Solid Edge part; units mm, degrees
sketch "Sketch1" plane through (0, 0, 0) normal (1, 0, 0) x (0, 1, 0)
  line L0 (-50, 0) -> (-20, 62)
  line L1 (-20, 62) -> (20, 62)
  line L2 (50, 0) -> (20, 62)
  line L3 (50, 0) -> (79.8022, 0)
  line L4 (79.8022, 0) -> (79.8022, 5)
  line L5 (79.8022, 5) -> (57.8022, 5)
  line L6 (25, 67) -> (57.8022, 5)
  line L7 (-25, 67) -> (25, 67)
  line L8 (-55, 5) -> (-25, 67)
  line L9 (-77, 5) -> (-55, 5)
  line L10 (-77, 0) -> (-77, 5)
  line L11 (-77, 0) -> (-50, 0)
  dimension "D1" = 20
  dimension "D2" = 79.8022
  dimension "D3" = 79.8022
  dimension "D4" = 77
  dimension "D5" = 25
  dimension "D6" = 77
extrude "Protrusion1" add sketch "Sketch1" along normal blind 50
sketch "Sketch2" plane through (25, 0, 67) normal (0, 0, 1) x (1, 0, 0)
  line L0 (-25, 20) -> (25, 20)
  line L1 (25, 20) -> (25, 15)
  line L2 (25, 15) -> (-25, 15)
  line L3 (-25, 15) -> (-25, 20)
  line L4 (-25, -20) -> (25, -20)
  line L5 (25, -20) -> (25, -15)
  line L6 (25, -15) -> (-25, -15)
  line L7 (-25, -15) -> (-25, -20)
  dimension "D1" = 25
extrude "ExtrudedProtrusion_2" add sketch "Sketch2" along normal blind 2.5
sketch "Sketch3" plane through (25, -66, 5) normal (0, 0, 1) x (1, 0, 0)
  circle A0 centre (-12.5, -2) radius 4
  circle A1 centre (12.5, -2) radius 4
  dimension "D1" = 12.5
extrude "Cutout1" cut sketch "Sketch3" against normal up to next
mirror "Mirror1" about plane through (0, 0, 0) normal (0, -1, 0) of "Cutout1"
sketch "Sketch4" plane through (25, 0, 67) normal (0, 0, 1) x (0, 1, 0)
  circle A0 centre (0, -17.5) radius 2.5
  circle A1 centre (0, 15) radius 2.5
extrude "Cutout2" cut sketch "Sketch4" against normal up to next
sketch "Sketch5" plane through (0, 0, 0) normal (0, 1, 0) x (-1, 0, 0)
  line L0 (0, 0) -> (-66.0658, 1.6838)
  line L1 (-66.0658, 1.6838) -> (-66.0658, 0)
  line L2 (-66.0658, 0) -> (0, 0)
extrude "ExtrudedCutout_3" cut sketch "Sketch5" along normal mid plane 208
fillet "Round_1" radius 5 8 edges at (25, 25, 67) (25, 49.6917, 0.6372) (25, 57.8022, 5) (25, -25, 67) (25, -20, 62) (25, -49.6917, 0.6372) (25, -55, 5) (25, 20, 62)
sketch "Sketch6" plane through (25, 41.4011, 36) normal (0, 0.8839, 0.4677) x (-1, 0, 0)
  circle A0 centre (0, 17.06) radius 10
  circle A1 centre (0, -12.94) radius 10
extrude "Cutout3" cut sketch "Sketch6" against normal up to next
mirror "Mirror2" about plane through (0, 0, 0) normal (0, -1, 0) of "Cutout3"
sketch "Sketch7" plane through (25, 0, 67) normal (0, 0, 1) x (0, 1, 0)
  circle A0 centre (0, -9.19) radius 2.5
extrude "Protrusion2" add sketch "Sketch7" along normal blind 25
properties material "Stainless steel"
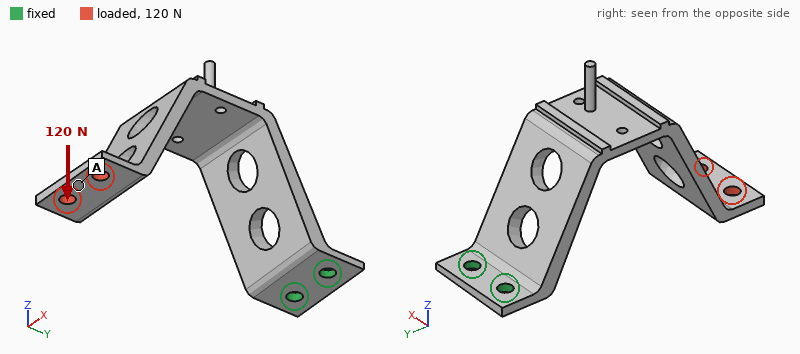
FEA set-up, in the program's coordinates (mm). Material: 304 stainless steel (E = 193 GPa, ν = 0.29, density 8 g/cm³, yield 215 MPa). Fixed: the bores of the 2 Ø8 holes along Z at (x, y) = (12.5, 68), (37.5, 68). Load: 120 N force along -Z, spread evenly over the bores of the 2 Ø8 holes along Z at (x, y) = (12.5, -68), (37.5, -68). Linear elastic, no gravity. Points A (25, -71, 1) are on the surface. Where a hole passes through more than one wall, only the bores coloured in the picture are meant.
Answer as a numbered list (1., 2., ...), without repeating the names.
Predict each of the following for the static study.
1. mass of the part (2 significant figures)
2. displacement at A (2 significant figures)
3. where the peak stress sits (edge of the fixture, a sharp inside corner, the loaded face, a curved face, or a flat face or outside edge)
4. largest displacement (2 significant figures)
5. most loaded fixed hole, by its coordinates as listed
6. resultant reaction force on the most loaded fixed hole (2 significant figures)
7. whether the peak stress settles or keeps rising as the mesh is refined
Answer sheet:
1. 510 g
2. 0.96 mm
3. edge of the fixture
4. 1.0 mm
5. (12.5, 68)
6. 100 N
7. keeps rising
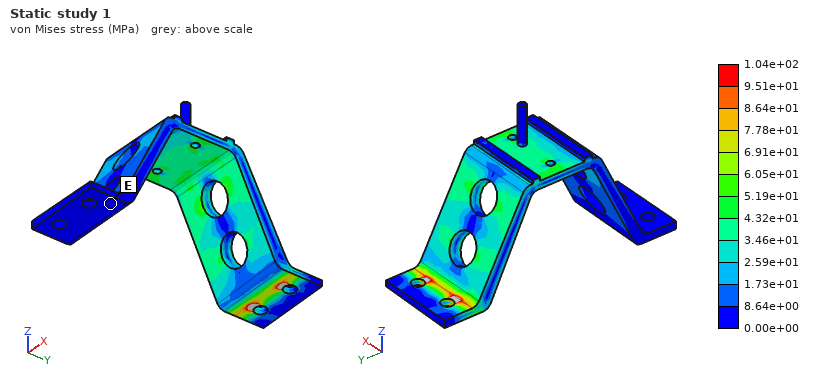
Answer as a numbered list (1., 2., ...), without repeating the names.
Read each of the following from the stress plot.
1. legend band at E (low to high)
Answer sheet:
1. 0.00e+00 to 8.64e+00 MPa
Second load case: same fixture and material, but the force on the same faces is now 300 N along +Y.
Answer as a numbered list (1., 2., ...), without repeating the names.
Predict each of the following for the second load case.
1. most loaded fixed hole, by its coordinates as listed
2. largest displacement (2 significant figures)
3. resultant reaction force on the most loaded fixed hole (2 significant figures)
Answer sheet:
1. (12.5, 68)
2. 1.3 mm
3. 160 N
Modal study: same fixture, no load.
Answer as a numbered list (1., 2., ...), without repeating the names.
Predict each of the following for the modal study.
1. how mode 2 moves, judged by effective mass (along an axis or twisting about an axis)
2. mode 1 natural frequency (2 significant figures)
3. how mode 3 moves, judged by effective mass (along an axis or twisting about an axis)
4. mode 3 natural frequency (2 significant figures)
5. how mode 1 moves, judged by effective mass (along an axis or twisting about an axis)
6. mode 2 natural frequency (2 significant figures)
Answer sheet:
1. along X
2. 160 Hz
3. along Y
4. 350 Hz
5. along Z
6. 290 Hz
